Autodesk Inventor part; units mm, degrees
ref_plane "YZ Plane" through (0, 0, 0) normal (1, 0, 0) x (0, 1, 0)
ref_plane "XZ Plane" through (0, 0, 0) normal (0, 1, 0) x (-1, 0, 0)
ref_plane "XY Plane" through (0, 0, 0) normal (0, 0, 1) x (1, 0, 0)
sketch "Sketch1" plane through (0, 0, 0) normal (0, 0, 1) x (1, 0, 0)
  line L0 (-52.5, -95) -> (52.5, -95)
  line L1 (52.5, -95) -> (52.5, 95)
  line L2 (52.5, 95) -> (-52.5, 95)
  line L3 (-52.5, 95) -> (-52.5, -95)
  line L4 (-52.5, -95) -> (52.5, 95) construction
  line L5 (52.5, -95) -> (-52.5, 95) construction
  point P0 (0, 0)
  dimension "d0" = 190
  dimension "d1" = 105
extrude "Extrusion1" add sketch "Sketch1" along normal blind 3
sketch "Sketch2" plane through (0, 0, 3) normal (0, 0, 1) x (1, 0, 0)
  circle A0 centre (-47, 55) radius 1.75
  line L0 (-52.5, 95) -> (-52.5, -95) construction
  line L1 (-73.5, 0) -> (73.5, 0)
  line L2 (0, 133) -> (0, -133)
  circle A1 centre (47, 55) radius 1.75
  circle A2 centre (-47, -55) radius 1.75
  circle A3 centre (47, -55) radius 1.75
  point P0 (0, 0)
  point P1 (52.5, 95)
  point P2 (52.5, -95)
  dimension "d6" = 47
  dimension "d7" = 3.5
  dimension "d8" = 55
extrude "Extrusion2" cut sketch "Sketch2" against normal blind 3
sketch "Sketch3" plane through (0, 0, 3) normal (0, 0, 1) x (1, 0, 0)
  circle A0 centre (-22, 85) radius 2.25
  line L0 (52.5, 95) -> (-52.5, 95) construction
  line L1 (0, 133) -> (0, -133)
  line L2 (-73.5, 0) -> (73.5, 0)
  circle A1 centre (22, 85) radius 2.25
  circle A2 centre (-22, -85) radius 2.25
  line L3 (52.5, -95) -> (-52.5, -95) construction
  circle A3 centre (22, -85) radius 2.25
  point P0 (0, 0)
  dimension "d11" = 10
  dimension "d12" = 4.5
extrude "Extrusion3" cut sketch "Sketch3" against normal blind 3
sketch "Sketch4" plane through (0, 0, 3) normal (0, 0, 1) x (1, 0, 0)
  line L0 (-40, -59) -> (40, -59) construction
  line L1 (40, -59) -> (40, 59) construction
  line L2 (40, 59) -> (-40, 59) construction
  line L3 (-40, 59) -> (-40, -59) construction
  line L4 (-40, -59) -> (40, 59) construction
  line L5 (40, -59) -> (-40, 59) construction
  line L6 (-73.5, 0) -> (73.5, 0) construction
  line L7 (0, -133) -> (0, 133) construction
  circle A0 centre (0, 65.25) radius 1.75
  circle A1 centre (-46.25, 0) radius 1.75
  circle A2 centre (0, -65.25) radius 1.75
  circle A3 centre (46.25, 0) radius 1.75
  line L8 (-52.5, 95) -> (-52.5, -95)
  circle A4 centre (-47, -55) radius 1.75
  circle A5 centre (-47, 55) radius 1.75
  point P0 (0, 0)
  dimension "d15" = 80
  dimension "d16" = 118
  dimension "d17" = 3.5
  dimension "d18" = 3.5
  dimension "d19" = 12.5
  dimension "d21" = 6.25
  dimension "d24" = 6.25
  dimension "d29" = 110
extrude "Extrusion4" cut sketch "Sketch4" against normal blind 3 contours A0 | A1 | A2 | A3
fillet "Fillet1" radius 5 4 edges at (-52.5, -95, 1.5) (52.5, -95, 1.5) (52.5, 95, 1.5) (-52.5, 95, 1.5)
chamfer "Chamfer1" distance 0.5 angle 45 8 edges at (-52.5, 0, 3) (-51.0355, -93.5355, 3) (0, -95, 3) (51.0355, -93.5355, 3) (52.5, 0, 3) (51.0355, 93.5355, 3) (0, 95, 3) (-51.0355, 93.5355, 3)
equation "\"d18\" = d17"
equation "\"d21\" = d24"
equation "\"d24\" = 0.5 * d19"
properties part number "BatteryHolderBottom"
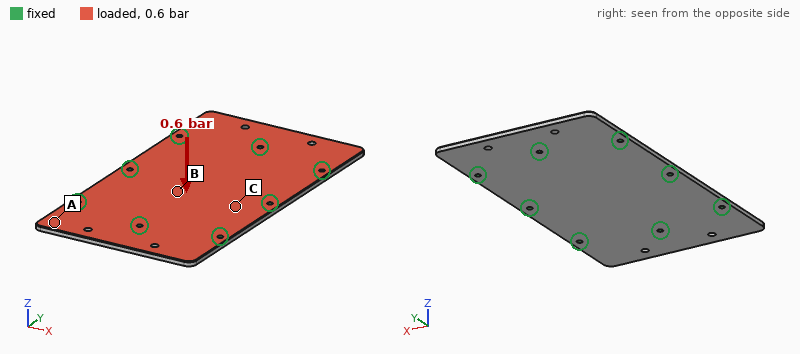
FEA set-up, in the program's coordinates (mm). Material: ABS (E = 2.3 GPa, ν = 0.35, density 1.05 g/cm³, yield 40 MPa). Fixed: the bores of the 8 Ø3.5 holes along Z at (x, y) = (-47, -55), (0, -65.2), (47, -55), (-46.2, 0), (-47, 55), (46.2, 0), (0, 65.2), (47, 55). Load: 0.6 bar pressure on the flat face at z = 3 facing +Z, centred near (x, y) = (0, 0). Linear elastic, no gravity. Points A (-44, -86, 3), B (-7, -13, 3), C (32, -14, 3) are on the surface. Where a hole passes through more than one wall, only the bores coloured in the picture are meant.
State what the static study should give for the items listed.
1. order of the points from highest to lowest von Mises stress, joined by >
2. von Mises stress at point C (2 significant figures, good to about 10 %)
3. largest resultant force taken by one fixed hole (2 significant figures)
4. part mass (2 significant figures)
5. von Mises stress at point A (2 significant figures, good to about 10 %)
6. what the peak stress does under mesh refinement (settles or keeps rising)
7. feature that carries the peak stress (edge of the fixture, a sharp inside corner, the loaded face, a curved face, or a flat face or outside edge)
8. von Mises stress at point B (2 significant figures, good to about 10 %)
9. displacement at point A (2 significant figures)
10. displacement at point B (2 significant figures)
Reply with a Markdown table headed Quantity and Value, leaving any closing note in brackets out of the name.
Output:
| Quantity | Value |
|---|---|
| order of the points from highest to lowest von Mises stress, joined by > | B > C > A |
| von Mises stress at point C | 6.7 MPa |
| largest resultant force taken by one fixed hole | 230 N |
| part mass | 62 g |
| von Mises stress at point A | 2.9 MPa |
| what the peak stress does under mesh refinement | keeps rising |
| feature that carries the peak stress | edge of the fixture |
| von Mises stress at point B | 11 MPa |
| displacement at point A | 1.6 mm |
| displacement at point B | 1.9 mm |
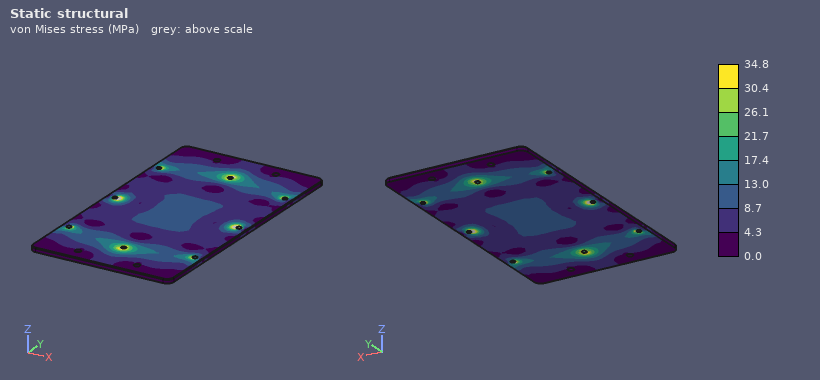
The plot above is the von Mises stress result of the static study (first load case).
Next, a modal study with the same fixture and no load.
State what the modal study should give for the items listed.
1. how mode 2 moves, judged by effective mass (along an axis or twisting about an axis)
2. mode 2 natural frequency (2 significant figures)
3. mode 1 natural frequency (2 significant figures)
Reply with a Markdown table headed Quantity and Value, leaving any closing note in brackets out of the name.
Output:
| Quantity | Value |
|---|---|
| how mode 2 moves, judged by effective mass | twisting about X |
| mode 2 natural frequency | 530 Hz |
| mode 1 natural frequency | 500 Hz |
